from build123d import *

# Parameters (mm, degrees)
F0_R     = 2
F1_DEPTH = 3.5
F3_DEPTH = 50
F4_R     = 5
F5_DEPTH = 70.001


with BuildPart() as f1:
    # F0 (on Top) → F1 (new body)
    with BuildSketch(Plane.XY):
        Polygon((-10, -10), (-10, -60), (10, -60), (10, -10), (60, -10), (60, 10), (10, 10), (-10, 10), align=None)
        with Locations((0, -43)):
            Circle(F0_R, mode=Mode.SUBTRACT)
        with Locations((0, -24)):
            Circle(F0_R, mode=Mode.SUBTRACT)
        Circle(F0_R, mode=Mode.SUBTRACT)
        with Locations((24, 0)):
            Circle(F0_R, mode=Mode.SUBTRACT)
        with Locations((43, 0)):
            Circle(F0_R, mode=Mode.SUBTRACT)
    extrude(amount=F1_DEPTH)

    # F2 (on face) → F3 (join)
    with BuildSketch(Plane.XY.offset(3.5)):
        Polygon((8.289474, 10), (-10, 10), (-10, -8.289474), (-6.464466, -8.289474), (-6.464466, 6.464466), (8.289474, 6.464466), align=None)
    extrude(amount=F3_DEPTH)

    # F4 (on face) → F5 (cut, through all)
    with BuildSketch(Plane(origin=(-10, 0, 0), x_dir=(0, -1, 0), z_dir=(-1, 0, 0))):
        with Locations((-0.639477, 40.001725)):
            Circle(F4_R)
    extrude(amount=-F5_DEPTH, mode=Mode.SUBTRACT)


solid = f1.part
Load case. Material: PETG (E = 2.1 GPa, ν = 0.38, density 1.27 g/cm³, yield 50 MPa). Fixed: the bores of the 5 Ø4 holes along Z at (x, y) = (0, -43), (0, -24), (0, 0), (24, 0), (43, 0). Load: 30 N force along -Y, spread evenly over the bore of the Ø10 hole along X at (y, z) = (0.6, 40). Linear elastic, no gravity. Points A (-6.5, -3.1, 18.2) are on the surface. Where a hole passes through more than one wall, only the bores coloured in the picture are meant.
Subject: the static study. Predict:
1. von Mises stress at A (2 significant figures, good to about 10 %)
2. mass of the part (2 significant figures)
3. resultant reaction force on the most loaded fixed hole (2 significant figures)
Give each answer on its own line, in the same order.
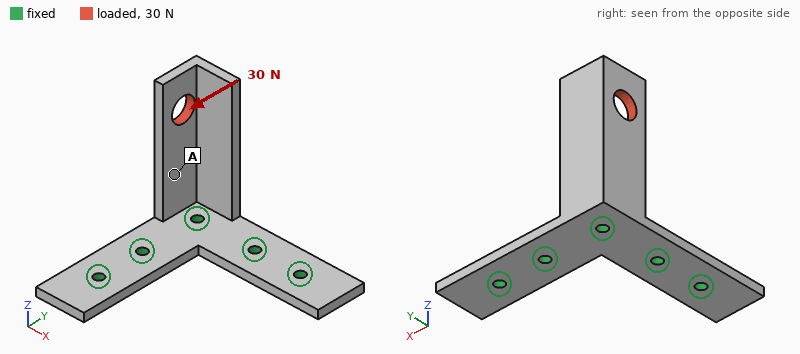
2.1 MPa
17 g
34 N
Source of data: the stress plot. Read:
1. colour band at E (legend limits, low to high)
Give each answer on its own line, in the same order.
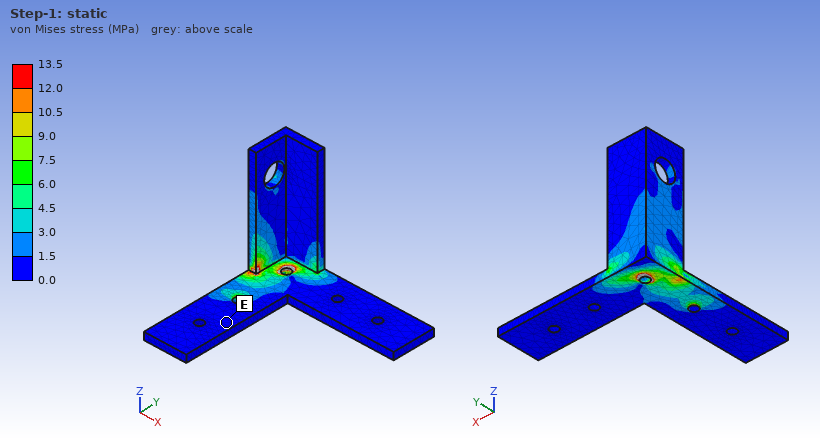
0.0 to 1.5 MPa
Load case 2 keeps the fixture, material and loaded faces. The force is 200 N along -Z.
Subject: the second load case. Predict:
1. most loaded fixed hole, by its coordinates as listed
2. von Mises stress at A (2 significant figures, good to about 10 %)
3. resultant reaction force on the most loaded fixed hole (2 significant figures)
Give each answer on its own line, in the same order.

(0, 0)
3.2 MPa
220 N
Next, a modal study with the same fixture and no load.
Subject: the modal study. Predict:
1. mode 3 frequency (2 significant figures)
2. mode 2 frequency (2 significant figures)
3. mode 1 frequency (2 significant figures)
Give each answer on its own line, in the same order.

1300 Hz
550 Hz
400 Hz
